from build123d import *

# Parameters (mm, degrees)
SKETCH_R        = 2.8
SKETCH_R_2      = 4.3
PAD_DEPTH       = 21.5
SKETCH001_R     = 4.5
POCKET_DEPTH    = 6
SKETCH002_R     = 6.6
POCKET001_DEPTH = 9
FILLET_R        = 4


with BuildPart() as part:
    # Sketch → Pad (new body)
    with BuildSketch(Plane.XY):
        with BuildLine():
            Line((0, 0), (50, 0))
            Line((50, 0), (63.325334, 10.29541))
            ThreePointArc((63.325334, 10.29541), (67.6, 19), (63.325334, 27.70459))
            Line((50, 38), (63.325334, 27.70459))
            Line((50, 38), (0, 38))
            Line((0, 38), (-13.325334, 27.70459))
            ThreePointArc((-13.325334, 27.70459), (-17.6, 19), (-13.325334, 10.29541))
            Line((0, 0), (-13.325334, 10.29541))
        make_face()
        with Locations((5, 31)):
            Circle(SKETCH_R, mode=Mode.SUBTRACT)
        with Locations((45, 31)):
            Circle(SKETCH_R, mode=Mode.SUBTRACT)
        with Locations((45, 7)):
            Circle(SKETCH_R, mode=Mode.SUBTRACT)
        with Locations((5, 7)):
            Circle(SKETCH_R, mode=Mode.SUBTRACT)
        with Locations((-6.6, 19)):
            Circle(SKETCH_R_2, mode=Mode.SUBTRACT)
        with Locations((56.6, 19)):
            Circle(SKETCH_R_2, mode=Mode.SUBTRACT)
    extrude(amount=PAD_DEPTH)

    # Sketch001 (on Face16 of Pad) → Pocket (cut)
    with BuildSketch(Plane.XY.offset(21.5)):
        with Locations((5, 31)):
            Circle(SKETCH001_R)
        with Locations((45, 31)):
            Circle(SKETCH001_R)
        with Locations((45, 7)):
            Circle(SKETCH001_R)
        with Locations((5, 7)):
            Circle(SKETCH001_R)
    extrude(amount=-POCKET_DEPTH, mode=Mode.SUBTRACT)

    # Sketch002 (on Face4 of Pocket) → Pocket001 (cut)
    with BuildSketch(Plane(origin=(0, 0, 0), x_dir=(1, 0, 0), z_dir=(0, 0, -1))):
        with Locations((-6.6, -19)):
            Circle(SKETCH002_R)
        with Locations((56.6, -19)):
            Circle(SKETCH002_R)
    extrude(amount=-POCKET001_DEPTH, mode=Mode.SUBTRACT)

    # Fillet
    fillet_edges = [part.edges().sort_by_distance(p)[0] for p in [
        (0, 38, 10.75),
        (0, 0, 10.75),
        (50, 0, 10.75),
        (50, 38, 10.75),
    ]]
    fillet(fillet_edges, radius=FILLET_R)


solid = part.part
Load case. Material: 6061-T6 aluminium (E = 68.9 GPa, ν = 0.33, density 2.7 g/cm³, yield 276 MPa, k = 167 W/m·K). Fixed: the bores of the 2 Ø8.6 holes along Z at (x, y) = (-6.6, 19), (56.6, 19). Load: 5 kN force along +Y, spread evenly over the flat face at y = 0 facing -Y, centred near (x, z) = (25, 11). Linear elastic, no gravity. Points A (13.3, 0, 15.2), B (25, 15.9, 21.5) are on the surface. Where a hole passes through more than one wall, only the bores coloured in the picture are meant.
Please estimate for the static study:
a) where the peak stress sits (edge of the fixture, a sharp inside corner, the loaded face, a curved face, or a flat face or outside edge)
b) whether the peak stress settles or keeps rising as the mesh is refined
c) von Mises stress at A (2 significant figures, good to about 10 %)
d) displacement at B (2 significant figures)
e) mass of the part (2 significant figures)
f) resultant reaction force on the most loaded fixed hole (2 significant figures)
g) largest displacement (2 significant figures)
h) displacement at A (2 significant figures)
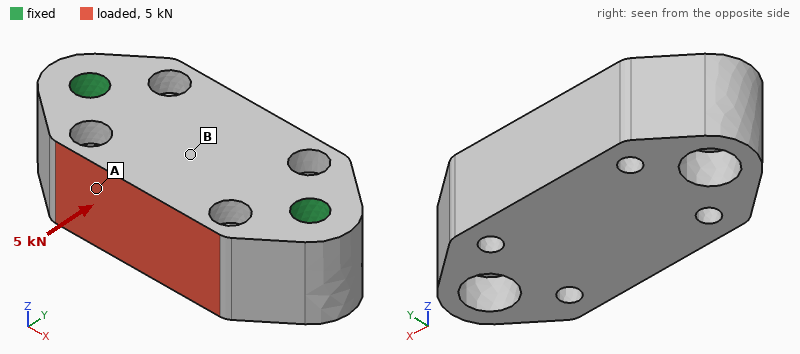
edge of the fixture
keeps rising
7.3 MPa
5.0 µm
140 g
2.5 kN
9.6 µm
6.5 µm
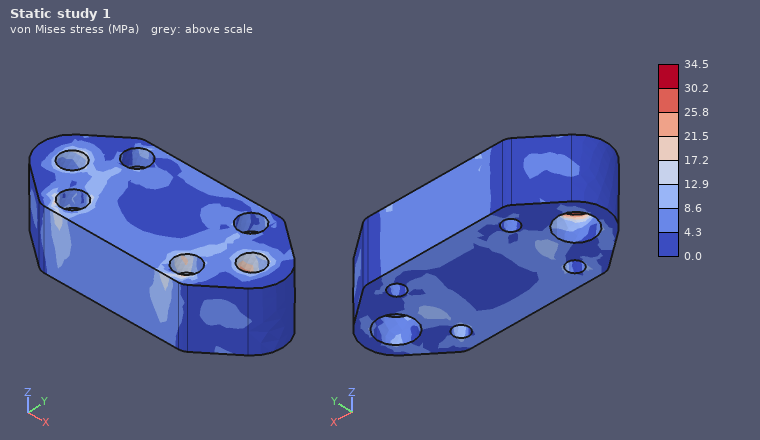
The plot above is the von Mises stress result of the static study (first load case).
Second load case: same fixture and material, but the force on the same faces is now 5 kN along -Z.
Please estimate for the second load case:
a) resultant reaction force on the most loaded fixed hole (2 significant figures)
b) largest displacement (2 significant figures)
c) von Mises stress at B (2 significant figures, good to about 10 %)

2.8 kN
37 µm
13 MPa
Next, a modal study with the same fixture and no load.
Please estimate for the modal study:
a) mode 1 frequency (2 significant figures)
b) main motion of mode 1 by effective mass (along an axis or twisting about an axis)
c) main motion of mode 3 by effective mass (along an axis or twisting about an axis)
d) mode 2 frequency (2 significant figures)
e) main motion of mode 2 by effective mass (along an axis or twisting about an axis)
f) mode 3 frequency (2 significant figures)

11 kHz
along Y
along Y
13 kHz
along Z
16 kHz
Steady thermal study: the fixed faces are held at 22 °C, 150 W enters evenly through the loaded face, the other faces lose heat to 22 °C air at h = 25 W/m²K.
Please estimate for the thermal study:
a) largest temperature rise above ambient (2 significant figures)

28 K
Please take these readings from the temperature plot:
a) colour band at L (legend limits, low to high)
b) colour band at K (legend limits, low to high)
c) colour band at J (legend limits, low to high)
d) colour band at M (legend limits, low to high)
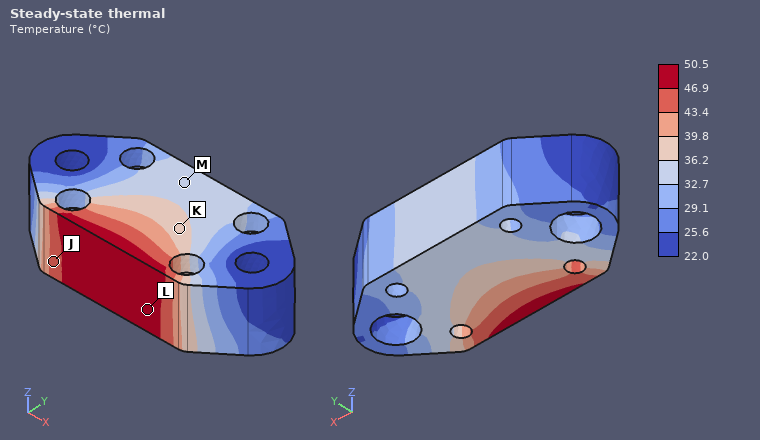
46.9 to 50.5 °C
36.2 to 39.8 °C
43.4 to 46.9 °C
32.7 to 36.2 °C
